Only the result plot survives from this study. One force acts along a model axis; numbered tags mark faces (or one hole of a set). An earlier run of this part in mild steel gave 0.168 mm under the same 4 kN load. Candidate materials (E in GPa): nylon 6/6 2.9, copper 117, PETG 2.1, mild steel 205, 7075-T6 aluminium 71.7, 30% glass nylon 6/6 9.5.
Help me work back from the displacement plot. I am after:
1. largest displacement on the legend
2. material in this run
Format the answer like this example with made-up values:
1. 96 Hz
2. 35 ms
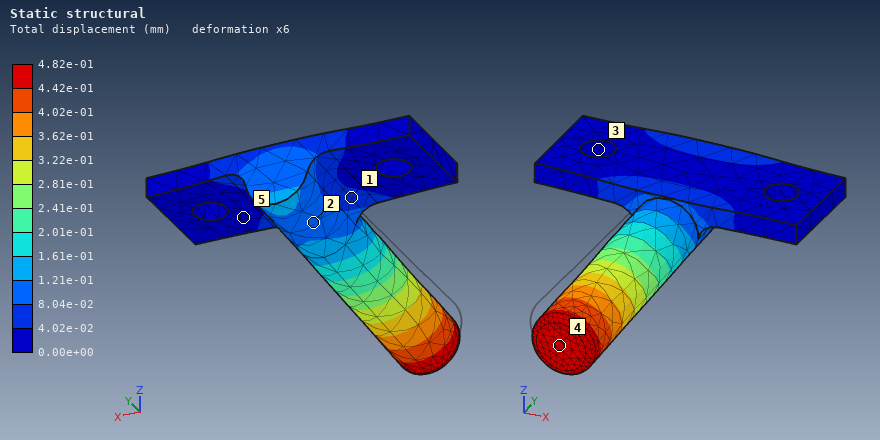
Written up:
1. 4.82e-01 mm
2. 7075-T6 aluminium
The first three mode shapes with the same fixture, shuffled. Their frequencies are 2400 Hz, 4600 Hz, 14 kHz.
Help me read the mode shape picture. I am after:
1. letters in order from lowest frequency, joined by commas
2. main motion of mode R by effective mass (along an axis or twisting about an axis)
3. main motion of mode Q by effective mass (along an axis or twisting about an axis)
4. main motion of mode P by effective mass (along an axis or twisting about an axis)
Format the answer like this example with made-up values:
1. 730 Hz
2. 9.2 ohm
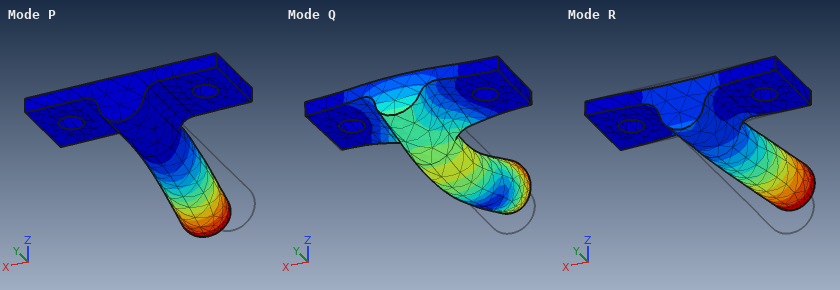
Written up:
1. R, P, Q
2. along Z
3. along Y
4. along X
